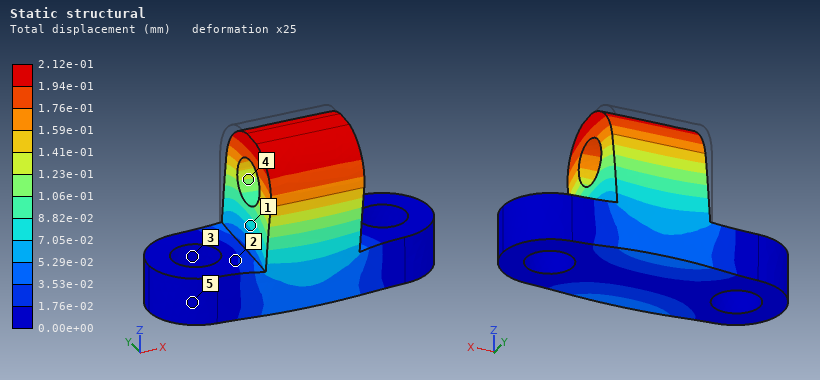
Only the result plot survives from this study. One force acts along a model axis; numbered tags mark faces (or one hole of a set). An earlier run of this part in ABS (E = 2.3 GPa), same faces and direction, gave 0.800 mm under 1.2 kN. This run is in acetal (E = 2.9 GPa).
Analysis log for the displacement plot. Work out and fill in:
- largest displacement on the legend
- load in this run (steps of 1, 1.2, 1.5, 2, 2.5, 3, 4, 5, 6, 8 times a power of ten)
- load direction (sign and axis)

2.12e-01 mm
400 N
-Y
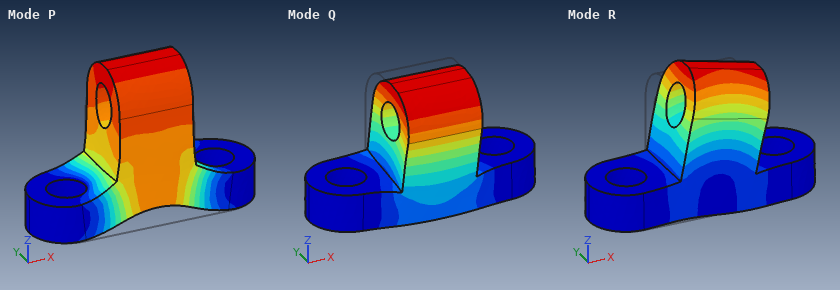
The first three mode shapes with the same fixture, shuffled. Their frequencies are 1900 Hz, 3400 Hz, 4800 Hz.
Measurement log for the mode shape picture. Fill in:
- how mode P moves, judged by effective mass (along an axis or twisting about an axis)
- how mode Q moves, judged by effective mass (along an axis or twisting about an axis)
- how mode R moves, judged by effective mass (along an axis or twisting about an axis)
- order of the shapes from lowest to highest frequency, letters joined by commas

along Z
along Y
along X
Q, R, P
